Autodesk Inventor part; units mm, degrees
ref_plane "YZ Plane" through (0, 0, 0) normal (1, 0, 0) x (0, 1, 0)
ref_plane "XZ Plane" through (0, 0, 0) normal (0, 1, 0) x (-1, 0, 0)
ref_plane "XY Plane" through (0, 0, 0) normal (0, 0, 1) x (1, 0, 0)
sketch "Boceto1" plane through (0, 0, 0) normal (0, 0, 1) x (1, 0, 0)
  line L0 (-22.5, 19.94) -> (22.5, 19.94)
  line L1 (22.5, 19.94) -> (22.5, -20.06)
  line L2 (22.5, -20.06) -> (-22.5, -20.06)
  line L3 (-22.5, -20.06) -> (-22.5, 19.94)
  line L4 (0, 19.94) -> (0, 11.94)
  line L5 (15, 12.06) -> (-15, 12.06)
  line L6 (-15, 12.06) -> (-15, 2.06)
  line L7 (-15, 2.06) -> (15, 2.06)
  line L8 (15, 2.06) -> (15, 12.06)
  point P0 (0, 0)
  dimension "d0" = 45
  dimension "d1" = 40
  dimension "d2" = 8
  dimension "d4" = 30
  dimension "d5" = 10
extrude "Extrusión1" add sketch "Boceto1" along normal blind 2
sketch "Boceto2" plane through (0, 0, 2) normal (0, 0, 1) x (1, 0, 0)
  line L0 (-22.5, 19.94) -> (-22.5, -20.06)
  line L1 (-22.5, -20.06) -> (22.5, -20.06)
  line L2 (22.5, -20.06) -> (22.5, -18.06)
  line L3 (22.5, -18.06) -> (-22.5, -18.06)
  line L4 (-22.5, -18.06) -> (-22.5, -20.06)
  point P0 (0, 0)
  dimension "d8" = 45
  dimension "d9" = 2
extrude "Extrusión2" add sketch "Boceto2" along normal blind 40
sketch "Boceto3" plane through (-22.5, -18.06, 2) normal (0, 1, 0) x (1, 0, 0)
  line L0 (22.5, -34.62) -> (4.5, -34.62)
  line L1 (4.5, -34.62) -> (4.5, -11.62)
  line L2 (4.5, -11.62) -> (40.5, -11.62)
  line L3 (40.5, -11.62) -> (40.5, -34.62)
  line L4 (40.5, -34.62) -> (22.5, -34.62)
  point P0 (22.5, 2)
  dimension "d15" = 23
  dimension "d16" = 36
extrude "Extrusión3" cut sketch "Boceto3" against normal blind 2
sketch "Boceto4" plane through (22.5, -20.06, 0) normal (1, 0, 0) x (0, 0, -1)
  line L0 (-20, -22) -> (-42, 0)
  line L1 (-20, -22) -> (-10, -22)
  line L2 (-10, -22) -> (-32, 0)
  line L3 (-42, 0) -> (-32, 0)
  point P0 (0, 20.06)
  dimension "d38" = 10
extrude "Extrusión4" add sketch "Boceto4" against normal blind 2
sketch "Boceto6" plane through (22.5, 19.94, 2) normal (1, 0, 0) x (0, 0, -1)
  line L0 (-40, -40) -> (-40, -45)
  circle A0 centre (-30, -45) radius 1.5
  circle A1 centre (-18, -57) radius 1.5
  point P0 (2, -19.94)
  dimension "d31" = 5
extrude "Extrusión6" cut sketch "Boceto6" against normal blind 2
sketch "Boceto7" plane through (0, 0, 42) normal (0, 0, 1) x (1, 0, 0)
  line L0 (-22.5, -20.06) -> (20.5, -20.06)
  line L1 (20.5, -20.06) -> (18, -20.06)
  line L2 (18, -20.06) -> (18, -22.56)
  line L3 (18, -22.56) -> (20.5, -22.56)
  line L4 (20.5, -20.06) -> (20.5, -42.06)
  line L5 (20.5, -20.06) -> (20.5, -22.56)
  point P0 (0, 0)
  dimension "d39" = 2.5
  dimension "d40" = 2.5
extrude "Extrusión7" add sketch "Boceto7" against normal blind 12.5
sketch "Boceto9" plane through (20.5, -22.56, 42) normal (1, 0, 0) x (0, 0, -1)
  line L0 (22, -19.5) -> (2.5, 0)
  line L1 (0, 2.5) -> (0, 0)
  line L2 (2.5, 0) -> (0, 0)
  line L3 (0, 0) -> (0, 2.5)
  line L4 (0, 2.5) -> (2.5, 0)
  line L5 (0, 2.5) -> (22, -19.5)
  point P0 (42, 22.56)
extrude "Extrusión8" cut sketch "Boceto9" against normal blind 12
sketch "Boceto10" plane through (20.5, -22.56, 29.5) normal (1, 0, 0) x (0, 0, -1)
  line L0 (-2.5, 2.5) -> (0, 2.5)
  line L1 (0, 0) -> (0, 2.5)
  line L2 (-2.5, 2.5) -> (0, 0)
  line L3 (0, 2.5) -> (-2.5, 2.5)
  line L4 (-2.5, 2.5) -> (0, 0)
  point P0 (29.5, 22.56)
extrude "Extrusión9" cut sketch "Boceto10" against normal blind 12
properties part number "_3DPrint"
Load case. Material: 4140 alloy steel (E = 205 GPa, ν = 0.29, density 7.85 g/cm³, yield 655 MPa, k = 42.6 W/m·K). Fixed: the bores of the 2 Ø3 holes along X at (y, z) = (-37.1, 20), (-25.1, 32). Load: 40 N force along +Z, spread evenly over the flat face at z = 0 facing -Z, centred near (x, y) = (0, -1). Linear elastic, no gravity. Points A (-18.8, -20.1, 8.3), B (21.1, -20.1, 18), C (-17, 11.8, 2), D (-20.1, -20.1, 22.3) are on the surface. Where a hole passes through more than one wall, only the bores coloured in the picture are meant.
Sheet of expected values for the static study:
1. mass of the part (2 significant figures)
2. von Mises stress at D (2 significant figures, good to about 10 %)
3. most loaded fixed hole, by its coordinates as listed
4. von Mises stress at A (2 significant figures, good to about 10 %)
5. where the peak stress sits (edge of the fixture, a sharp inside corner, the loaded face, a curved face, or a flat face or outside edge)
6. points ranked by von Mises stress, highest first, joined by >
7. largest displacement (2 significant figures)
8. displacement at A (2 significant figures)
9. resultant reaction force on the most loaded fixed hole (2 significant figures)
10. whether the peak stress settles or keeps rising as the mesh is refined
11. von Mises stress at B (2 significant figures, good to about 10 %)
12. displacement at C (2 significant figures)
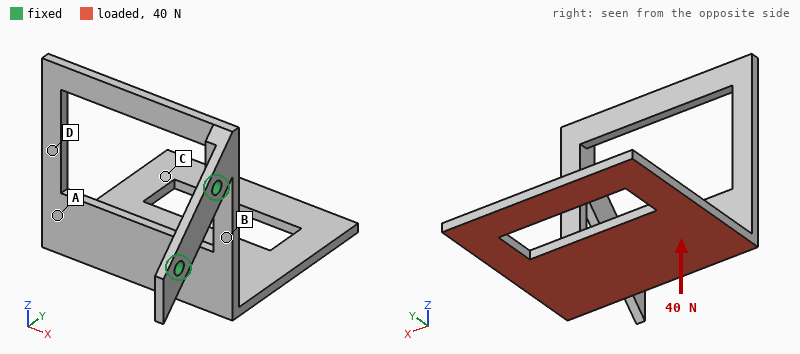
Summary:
43 g
82 MPa
(-25.1, 32)
37 MPa
edge of the fixture
B > D > A > C
1.0 mm
0.38 mm
50 N
keeps rising
150 MPa
0.85 mm
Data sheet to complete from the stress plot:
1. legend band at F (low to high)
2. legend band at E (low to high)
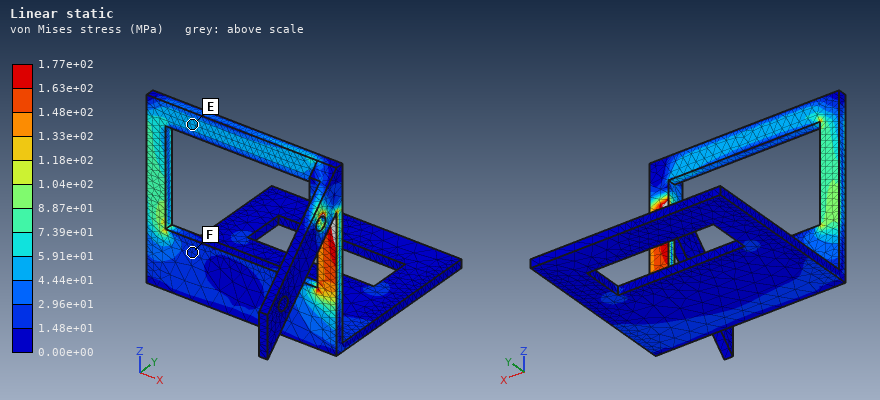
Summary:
1.48e+01 to 2.96e+01 MPa
4.44e+01 to 5.91e+01 MPa
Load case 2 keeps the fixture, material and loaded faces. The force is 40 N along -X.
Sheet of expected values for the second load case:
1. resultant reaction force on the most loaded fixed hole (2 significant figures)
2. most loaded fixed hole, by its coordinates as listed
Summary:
42 N
(-25.1, 32)
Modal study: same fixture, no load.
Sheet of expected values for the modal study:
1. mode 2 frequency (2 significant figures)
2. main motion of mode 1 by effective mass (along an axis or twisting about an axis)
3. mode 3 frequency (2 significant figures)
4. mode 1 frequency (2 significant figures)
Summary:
280 Hz
along Y
540 Hz
160 Hz
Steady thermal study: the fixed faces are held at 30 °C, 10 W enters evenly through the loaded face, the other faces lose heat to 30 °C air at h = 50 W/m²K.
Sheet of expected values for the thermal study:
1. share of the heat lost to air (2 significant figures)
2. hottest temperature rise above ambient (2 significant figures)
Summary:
95 %
72 K
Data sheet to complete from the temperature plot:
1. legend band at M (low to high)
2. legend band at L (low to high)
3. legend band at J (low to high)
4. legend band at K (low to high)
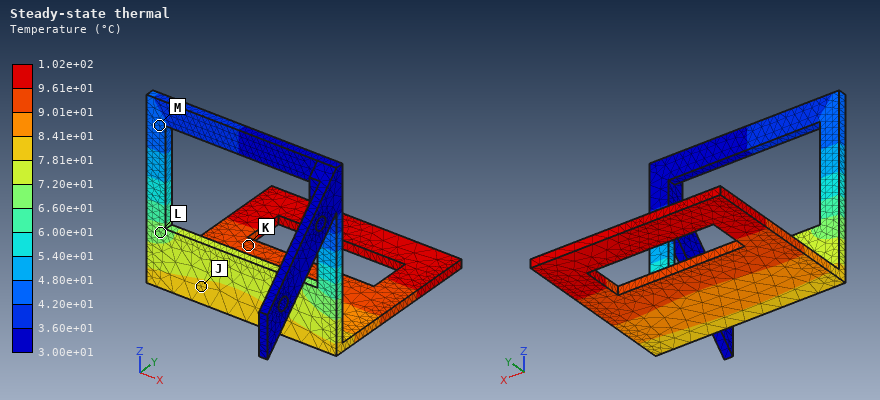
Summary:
4.20e+01 to 4.80e+01 °C
6.60e+01 to 7.20e+01 °C
7.81e+01 to 8.41e+01 °C
9.01e+01 to 9.61e+01 °C
